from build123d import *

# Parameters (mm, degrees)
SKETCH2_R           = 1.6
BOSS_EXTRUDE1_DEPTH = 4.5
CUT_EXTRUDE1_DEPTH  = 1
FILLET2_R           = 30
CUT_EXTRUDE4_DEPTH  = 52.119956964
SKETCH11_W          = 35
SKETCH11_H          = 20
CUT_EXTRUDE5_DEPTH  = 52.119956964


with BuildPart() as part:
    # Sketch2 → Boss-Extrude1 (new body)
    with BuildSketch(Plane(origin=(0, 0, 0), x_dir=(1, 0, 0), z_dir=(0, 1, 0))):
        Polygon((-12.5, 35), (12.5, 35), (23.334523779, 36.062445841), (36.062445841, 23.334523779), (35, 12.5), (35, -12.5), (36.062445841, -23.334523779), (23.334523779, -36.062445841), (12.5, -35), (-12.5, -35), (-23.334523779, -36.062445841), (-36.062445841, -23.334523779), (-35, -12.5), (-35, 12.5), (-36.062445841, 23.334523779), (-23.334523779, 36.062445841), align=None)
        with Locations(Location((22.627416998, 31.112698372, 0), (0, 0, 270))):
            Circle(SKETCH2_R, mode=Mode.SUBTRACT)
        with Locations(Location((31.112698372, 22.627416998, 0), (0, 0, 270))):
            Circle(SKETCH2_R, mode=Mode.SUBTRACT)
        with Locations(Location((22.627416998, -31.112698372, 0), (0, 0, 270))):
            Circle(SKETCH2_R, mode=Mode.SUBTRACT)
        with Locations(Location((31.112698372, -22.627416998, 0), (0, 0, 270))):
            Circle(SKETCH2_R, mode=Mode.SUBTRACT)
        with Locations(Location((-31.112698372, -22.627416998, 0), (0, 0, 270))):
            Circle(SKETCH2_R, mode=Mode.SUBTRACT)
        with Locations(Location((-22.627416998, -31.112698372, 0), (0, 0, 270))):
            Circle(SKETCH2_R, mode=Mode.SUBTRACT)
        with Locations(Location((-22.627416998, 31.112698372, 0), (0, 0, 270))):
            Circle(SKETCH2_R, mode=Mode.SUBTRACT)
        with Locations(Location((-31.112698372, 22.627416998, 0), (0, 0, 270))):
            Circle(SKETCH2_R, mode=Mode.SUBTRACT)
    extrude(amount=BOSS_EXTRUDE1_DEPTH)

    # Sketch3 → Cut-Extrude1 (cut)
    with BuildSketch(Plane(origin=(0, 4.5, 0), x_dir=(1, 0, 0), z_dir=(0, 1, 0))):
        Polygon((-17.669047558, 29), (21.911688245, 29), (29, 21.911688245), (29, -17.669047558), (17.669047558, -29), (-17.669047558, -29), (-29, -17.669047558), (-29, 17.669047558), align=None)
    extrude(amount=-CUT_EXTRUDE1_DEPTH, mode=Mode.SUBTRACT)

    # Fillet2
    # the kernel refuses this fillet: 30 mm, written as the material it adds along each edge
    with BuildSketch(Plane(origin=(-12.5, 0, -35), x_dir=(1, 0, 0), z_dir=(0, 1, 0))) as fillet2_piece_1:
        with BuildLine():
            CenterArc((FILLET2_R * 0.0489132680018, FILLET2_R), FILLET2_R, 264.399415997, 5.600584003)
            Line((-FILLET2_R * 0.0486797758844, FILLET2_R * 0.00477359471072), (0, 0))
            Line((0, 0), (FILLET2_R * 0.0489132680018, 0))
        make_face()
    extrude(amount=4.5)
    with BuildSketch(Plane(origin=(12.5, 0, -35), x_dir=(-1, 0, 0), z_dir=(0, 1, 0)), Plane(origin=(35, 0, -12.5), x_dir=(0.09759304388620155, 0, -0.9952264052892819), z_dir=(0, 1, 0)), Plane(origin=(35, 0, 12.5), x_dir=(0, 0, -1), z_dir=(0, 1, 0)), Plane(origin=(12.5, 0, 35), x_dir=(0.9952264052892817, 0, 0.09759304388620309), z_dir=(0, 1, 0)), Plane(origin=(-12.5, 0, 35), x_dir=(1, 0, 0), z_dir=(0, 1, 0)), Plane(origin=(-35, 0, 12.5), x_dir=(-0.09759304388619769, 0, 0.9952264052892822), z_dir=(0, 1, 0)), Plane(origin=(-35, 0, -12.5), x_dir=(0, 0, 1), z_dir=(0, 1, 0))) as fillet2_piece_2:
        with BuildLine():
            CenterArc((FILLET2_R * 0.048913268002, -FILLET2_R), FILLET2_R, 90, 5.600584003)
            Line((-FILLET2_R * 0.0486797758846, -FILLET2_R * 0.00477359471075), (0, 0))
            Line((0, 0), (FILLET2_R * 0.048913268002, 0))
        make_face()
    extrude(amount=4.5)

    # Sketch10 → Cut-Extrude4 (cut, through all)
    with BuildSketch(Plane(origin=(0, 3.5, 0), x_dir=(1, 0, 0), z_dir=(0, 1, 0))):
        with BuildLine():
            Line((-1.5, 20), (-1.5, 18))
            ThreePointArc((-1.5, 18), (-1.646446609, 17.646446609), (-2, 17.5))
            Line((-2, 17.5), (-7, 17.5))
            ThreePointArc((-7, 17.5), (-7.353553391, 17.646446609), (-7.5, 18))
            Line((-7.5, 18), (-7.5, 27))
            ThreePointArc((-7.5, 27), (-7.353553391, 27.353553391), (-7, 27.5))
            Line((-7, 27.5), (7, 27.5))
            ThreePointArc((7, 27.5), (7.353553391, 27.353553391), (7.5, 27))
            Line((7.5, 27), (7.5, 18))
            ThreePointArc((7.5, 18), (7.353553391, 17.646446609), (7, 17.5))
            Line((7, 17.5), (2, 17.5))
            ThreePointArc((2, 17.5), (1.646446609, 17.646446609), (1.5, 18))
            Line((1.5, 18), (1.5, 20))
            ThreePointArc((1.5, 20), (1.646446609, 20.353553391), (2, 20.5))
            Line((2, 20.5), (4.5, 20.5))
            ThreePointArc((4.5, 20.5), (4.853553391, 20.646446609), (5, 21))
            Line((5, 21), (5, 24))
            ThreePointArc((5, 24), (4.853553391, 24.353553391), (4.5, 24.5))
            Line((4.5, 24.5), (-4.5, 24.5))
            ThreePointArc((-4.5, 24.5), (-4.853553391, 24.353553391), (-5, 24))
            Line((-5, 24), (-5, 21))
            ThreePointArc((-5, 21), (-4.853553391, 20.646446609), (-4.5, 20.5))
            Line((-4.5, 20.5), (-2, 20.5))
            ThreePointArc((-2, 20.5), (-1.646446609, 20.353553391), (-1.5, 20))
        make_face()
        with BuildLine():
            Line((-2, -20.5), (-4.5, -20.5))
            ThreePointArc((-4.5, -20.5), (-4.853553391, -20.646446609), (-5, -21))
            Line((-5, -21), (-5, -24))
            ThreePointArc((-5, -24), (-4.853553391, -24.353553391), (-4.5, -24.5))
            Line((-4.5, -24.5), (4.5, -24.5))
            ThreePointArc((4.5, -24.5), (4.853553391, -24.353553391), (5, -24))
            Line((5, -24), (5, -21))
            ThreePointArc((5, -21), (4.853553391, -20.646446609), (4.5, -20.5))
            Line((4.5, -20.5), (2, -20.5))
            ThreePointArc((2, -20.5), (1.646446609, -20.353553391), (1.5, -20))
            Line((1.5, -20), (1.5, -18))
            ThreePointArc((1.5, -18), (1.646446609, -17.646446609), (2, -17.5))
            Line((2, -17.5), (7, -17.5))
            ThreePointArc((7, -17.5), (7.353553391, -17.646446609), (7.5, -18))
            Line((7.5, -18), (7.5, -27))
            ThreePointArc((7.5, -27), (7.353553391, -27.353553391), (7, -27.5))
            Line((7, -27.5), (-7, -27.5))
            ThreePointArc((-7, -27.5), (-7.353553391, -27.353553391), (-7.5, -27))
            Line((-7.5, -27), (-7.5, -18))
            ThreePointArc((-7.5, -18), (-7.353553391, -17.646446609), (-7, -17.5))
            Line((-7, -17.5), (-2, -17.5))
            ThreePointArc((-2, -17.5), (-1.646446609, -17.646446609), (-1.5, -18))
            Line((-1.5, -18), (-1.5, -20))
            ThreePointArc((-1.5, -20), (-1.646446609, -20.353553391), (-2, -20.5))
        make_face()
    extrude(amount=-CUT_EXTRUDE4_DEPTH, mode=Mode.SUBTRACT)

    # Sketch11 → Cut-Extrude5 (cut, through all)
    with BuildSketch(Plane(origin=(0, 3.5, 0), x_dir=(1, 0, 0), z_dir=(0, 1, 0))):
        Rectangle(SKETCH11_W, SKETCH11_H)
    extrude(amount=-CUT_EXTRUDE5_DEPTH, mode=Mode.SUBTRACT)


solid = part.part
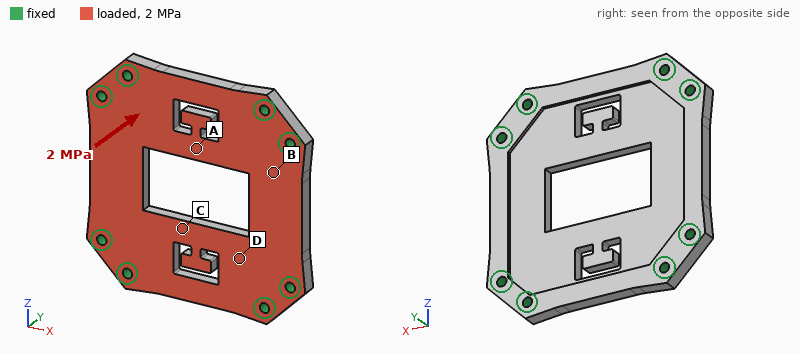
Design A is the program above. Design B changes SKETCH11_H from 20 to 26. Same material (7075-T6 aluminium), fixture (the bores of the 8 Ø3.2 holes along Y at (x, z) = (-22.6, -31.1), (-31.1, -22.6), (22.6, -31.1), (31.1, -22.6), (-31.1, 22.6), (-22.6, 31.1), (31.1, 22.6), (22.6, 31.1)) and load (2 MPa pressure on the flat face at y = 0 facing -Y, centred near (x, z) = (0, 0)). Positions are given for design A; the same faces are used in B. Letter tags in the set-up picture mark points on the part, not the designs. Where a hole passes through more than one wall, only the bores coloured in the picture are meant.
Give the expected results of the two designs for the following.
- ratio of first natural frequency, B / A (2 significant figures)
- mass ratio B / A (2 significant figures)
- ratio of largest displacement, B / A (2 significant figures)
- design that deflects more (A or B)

1.1
0.95
0.78
A
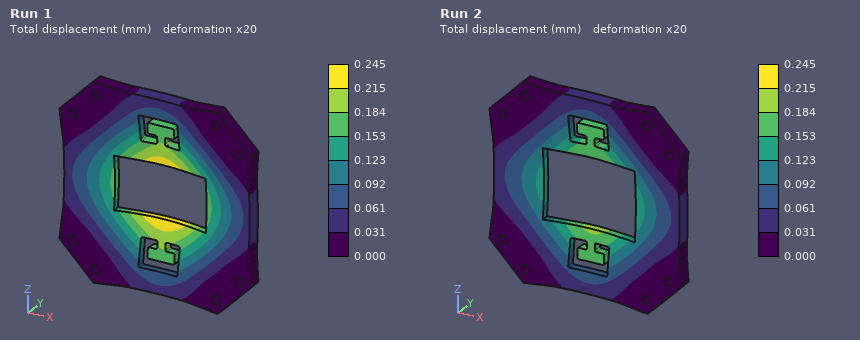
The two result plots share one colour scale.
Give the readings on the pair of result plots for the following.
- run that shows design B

Run 2
